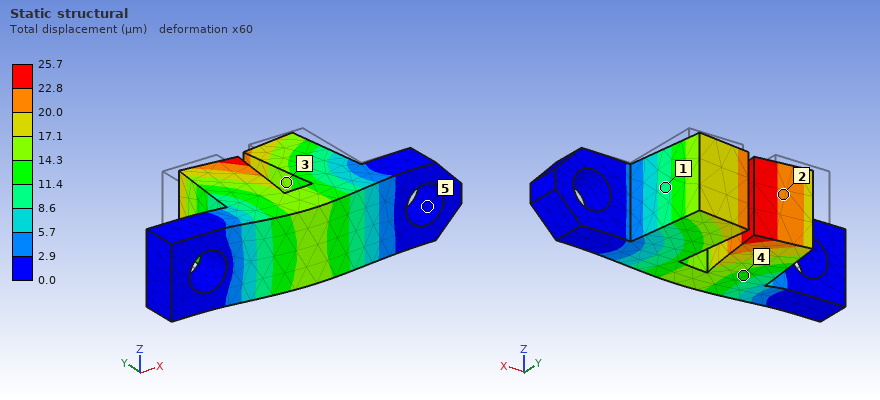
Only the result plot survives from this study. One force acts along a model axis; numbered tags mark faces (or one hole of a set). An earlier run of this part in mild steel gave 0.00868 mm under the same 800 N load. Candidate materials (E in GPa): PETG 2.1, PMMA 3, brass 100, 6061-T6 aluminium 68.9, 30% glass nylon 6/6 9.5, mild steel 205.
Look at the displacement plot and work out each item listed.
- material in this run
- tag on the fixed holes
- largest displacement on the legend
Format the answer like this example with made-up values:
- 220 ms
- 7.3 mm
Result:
- 6061-T6 aluminium
- 5
- 25.7 µm
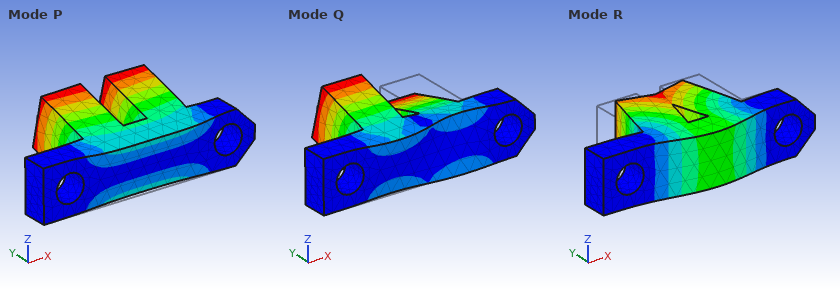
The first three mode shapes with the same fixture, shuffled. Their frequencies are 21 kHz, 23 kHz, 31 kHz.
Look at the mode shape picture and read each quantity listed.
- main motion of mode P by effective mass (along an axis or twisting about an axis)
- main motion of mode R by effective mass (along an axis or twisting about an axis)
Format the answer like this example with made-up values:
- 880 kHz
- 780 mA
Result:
- along Z
- along Y
